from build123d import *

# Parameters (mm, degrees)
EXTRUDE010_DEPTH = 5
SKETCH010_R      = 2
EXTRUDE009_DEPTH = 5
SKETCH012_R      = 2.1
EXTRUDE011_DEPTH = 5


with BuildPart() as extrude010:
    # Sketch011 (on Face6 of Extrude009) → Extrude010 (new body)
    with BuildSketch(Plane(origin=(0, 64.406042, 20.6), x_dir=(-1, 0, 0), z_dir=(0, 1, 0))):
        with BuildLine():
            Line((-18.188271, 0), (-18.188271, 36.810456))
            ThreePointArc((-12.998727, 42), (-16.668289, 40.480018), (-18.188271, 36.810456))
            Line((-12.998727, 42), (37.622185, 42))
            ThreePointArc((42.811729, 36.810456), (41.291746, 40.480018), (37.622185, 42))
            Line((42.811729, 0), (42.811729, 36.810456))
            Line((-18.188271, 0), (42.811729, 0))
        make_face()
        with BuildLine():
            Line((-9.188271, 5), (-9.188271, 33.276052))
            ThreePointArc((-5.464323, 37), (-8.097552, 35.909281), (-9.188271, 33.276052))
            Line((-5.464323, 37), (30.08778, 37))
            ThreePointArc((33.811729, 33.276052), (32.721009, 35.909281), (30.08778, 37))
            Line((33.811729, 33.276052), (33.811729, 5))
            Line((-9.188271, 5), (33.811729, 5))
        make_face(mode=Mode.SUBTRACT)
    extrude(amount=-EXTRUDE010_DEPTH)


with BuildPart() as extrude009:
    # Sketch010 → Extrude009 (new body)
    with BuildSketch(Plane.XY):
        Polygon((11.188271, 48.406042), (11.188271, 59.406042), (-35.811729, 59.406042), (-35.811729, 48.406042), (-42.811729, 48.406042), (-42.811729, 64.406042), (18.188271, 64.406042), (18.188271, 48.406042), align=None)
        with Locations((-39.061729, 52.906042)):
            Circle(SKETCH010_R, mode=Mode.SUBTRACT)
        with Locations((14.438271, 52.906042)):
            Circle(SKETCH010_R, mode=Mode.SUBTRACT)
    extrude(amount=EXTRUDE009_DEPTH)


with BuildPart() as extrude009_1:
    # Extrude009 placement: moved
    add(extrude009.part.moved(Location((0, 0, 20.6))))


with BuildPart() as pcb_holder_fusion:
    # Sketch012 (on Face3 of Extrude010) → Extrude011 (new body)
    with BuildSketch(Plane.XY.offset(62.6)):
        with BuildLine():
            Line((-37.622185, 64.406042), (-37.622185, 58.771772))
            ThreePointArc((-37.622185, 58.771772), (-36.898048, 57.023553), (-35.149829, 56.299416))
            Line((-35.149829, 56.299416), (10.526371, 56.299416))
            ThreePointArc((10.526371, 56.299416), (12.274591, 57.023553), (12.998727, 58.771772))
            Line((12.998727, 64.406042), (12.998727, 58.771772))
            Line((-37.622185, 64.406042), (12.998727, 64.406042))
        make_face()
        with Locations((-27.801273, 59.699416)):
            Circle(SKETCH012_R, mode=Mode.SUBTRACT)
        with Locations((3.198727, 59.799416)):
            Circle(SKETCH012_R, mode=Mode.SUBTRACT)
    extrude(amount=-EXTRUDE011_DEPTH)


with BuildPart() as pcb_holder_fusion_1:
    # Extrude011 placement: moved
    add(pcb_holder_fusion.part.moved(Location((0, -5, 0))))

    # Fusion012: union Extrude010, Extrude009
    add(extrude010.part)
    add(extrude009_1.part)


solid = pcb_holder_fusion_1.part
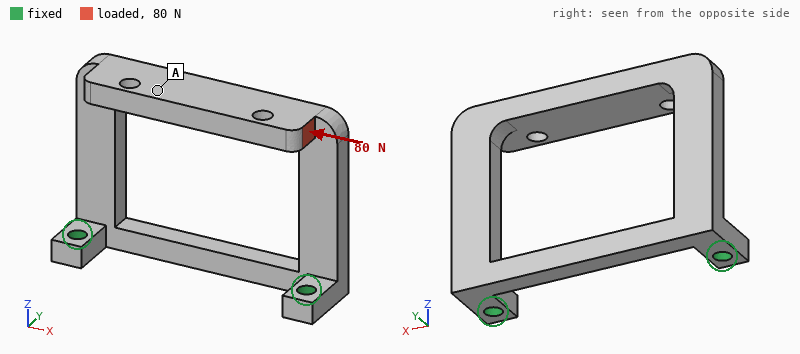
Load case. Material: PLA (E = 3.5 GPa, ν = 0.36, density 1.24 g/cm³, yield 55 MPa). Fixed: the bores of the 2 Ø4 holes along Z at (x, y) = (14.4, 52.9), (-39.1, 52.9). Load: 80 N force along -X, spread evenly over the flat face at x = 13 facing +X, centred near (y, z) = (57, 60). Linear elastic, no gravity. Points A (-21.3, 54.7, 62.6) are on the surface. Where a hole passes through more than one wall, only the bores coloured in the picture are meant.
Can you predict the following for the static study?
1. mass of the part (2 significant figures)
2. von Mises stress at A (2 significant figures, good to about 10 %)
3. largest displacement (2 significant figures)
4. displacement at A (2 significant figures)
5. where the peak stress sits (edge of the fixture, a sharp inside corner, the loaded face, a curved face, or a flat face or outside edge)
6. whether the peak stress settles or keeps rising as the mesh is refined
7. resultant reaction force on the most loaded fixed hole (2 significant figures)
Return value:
10 g
3.2 MPa
0.78 mm
0.68 mm
edge of the fixture
keeps rising
57 N
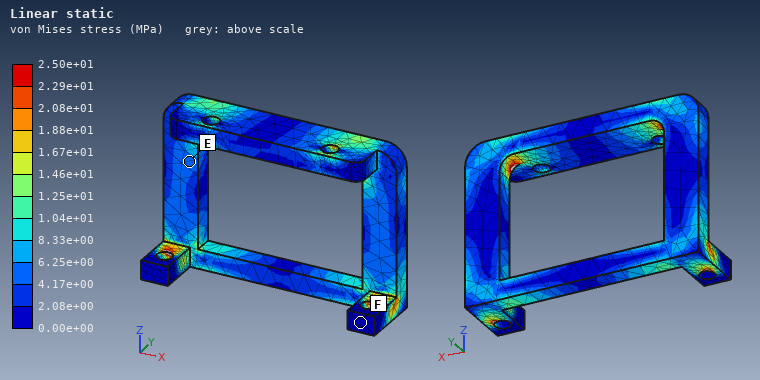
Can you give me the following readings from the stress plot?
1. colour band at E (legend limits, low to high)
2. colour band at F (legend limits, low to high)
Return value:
4.17e+00 to 6.25e+00 MPa
0.00e+00 to 2.08e+00 MPa
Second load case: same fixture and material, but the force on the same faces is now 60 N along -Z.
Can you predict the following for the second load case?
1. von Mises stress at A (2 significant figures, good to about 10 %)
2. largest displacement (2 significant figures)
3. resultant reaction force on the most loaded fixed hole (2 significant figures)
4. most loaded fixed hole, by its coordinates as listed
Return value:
1.8 MPa
0.52 mm
58 N
(14.4, 52.9)
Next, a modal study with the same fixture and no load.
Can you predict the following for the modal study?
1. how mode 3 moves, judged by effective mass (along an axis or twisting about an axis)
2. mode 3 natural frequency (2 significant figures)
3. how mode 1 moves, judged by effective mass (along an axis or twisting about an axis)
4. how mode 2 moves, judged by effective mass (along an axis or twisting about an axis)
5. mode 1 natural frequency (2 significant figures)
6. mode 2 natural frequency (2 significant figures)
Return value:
along X
910 Hz
along Y
along X
340 Hz
730 Hz
